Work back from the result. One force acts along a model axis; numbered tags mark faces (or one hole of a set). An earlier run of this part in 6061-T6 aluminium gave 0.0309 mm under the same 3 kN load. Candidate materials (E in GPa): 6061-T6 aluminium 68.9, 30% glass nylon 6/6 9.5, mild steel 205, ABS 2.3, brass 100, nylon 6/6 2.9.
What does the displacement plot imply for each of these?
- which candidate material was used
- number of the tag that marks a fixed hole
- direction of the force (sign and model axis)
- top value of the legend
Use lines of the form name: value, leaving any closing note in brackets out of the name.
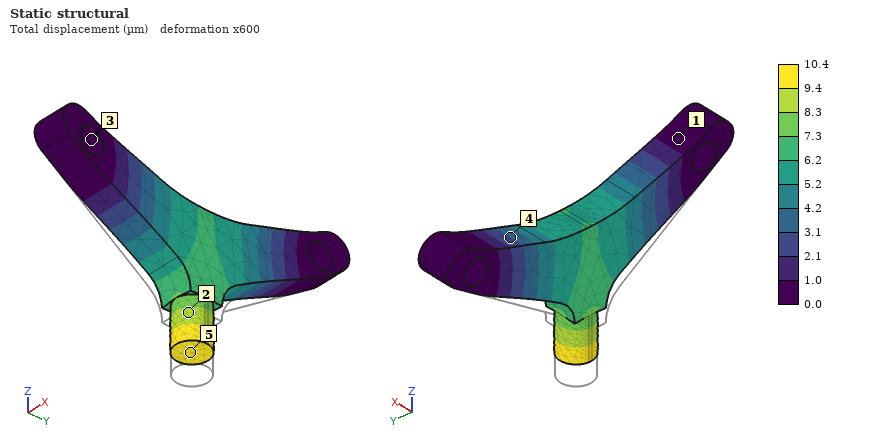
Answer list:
which candidate material was used: mild steel
number of the tag that marks a fixed hole: 3
direction of the force: +Z
top value of the legend: 10.4 µm
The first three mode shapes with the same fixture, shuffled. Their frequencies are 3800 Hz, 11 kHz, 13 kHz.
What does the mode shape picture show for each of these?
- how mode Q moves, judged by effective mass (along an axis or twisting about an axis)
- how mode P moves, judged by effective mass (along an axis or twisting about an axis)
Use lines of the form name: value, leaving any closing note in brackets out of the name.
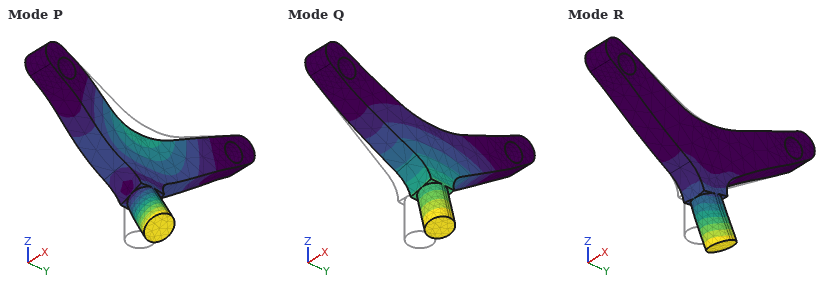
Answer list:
how mode Q moves, judged by effective mass: along X
how mode P moves, judged by effective mass: along X
